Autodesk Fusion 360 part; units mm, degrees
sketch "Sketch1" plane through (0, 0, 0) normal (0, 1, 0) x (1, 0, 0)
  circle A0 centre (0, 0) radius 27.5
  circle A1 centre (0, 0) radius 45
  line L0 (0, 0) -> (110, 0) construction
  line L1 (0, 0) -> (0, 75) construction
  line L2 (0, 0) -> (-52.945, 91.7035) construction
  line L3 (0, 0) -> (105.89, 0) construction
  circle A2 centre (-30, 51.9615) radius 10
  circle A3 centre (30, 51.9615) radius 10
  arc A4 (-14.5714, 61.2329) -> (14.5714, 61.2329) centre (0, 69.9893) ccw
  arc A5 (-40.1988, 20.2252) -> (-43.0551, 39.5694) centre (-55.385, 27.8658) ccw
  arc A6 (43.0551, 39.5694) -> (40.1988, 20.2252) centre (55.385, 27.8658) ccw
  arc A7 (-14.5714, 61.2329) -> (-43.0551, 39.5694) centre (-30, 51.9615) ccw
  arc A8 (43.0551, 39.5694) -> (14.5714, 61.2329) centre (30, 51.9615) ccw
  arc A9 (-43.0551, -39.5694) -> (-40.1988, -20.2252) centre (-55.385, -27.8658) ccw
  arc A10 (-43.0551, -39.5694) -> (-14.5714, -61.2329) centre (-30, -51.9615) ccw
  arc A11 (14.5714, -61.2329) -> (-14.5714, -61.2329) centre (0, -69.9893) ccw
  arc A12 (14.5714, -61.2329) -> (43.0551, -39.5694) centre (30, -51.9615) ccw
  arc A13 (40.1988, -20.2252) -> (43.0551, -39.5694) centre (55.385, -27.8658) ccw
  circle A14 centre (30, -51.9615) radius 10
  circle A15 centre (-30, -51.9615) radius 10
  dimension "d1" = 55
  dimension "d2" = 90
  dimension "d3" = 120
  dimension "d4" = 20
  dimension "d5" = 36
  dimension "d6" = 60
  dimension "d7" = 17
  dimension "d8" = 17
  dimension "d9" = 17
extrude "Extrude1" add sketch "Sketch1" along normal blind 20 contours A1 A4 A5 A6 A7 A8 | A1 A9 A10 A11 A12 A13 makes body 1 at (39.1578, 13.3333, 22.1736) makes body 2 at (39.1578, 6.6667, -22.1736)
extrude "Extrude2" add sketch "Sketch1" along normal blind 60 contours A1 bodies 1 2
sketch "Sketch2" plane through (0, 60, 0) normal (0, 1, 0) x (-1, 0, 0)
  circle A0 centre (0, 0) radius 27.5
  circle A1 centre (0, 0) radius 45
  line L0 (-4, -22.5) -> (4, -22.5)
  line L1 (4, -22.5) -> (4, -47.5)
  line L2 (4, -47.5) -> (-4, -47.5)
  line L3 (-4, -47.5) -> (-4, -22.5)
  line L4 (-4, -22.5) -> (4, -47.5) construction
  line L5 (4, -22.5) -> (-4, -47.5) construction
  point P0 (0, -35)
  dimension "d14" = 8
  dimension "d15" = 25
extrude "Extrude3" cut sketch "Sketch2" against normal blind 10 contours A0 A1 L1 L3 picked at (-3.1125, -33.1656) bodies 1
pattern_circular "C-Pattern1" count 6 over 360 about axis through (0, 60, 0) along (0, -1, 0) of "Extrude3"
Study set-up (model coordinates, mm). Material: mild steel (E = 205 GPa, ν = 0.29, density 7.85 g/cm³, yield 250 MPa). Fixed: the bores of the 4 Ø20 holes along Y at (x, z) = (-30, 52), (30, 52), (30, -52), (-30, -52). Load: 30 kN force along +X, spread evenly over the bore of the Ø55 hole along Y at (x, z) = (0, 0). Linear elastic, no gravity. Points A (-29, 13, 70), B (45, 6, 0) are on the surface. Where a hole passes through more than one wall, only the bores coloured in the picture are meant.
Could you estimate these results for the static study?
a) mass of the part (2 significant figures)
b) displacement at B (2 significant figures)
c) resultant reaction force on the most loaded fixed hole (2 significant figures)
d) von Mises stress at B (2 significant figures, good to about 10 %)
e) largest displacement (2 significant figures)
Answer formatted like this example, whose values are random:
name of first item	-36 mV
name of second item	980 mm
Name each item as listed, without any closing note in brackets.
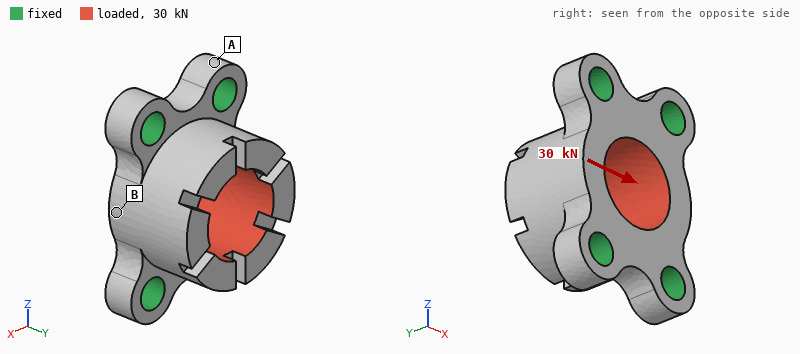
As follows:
mass of the part	2.3 kg
displacement at B	5.2 µm
resultant reaction force on the most loaded fixed hole	9.3 kN
von Mises stress at B	9.4 MPa
largest displacement	12 µm
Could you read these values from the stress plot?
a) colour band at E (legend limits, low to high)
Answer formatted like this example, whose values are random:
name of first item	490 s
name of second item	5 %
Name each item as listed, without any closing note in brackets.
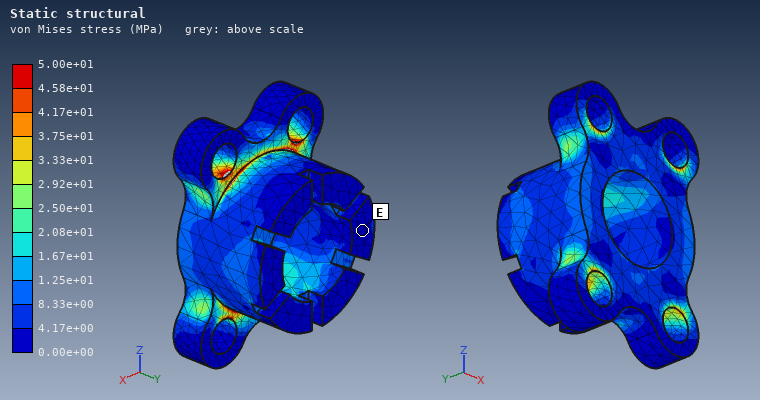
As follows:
colour band at E	0.00e+00 to 4.17e+00 MPa
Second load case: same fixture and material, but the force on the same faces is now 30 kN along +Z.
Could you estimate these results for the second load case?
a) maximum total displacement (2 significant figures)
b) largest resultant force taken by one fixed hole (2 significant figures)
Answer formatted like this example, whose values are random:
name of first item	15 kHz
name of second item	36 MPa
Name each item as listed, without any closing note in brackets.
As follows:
maximum total displacement	6.8 µm
largest resultant force taken by one fixed hole	8.3 kN
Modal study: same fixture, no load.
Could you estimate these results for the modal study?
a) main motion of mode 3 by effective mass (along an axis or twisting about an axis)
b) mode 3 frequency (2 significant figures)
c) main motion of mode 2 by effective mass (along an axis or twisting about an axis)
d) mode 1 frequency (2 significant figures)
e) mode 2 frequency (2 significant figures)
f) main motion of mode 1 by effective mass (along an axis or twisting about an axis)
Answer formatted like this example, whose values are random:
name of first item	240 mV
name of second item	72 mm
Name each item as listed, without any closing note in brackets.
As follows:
main motion of mode 3 by effective mass	along Z
mode 3 frequency	10 kHz
main motion of mode 2 by effective mass	along Y
mode 1 frequency	6800 Hz
mode 2 frequency	7900 Hz
main motion of mode 1 by effective mass	along X
